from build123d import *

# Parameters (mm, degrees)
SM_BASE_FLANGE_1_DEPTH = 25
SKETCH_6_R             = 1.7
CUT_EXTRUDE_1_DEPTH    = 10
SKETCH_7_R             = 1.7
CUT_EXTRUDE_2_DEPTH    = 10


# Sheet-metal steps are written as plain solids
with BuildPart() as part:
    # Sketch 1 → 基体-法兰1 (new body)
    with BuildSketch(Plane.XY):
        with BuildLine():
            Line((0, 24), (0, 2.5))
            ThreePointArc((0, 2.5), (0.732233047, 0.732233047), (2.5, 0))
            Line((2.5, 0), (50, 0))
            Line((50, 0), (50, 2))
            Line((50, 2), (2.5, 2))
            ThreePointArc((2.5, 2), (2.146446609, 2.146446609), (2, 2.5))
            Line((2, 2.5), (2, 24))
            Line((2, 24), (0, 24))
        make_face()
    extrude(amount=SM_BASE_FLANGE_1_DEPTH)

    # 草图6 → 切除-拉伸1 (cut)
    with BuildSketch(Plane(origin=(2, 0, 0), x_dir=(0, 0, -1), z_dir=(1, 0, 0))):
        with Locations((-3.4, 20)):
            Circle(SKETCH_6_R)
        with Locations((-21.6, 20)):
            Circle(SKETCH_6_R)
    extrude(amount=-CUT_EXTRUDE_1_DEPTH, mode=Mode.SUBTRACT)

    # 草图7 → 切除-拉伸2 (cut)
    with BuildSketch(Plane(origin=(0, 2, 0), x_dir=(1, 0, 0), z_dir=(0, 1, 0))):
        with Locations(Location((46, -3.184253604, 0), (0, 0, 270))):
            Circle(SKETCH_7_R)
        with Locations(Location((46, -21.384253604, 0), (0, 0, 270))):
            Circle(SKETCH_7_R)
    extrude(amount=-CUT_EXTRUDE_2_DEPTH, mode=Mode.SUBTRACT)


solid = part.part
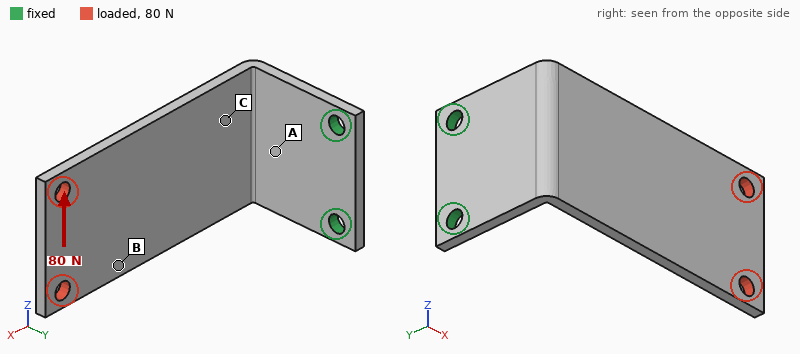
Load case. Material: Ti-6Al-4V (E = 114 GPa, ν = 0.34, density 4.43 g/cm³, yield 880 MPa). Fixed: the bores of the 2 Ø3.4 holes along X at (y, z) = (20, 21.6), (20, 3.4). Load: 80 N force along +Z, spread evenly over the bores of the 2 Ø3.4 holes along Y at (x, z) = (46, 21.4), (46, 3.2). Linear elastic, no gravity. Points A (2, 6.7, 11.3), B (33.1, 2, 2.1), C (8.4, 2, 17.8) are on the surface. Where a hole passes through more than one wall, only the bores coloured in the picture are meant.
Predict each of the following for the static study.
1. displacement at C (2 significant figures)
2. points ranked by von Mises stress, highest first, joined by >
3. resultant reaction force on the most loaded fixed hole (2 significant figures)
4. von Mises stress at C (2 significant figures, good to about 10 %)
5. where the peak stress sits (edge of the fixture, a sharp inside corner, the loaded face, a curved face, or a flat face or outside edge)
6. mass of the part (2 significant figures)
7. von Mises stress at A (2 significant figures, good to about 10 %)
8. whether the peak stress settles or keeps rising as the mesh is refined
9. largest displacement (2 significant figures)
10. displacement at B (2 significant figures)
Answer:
0.12 mm
A > C > B
210 N
42 MPa
edge of the fixture
15 g
130 MPa
keeps rising
0.65 mm
0.43 mm
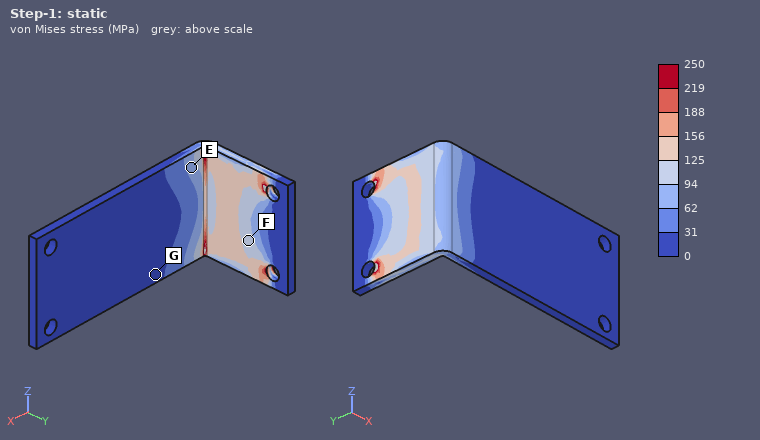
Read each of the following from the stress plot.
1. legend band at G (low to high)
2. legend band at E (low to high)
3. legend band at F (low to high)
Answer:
0 to 31 MPa
62 to 94 MPa
94 to 125 MPa
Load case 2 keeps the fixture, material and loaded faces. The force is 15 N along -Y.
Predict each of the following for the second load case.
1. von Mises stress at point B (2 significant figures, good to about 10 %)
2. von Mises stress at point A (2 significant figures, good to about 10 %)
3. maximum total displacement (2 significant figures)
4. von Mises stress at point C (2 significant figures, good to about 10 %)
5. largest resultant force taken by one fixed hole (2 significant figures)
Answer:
12 MPa
38 MPa
0.56 mm
31 MPa
9.0 N
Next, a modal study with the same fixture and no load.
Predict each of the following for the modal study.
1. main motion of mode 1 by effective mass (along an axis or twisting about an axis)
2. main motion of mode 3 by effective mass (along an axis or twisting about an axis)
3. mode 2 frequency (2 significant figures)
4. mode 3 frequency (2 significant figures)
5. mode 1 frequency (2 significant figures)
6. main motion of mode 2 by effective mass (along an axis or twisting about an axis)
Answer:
along Y
along X
890 Hz
1900 Hz
440 Hz
along Z
